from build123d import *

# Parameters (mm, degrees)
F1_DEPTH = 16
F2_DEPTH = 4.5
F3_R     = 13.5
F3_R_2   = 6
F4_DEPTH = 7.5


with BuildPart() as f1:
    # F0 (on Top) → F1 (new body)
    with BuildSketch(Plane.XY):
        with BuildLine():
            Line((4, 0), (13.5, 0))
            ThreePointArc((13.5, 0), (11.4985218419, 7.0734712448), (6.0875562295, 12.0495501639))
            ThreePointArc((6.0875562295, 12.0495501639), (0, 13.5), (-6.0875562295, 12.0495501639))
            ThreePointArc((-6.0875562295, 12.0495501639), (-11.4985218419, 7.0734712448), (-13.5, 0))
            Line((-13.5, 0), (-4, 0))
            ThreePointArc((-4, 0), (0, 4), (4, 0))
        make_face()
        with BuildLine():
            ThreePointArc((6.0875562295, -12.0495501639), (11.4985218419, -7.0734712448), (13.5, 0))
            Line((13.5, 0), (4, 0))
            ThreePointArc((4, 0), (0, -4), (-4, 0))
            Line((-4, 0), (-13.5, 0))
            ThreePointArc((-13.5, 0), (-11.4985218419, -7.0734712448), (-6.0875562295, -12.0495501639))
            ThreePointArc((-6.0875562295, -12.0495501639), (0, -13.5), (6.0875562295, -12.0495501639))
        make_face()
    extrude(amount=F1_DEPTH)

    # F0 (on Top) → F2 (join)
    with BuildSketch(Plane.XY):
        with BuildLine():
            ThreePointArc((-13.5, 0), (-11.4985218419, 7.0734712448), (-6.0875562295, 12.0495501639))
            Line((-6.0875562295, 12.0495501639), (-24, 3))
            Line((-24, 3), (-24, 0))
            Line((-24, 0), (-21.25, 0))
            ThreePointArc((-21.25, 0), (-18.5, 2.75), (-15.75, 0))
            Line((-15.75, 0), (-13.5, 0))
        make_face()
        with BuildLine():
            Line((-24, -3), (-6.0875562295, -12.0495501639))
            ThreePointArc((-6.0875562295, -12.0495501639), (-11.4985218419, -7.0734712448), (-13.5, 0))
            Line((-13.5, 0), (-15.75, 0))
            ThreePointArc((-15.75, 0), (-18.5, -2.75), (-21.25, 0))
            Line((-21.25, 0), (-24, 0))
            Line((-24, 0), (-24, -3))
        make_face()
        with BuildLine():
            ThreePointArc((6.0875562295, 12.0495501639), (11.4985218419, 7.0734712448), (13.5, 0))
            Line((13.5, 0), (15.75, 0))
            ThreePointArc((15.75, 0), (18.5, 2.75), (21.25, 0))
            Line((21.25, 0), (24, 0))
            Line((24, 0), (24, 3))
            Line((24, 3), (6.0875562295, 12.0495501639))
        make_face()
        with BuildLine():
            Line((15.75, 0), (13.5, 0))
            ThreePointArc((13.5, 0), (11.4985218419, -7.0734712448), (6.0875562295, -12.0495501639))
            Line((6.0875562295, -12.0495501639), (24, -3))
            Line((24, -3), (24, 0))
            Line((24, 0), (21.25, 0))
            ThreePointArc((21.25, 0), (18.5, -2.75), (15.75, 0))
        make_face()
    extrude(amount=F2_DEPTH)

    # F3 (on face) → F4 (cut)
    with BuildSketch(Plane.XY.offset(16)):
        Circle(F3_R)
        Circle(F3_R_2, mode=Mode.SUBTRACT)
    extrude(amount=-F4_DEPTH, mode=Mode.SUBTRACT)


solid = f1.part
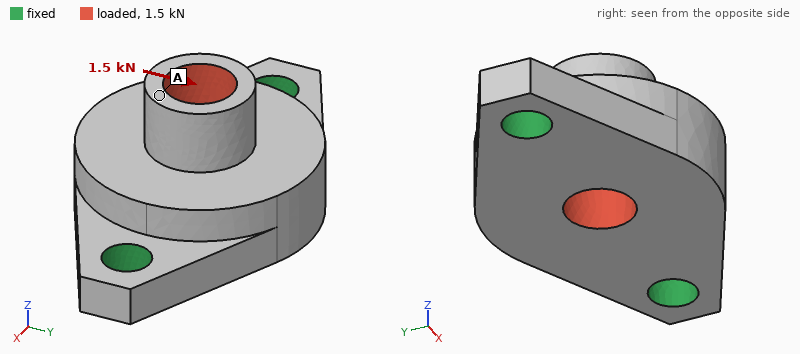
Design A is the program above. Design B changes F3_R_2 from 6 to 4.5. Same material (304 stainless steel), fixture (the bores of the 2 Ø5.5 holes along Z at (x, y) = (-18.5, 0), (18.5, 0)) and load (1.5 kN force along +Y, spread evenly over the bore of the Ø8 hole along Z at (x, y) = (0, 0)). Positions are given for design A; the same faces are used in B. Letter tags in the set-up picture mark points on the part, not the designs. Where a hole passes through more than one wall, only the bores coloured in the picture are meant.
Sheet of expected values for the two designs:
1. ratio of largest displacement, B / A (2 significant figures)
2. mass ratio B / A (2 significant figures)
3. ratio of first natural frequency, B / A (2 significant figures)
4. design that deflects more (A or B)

1.5
0.94
1.1
B
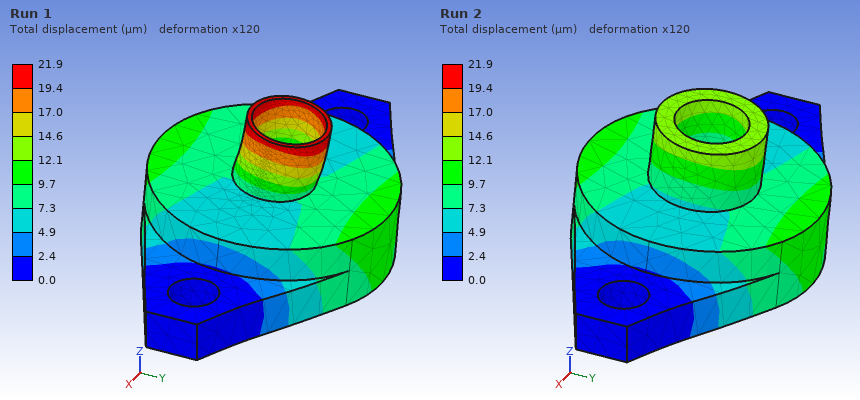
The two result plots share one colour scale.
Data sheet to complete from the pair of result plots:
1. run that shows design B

Run 1
